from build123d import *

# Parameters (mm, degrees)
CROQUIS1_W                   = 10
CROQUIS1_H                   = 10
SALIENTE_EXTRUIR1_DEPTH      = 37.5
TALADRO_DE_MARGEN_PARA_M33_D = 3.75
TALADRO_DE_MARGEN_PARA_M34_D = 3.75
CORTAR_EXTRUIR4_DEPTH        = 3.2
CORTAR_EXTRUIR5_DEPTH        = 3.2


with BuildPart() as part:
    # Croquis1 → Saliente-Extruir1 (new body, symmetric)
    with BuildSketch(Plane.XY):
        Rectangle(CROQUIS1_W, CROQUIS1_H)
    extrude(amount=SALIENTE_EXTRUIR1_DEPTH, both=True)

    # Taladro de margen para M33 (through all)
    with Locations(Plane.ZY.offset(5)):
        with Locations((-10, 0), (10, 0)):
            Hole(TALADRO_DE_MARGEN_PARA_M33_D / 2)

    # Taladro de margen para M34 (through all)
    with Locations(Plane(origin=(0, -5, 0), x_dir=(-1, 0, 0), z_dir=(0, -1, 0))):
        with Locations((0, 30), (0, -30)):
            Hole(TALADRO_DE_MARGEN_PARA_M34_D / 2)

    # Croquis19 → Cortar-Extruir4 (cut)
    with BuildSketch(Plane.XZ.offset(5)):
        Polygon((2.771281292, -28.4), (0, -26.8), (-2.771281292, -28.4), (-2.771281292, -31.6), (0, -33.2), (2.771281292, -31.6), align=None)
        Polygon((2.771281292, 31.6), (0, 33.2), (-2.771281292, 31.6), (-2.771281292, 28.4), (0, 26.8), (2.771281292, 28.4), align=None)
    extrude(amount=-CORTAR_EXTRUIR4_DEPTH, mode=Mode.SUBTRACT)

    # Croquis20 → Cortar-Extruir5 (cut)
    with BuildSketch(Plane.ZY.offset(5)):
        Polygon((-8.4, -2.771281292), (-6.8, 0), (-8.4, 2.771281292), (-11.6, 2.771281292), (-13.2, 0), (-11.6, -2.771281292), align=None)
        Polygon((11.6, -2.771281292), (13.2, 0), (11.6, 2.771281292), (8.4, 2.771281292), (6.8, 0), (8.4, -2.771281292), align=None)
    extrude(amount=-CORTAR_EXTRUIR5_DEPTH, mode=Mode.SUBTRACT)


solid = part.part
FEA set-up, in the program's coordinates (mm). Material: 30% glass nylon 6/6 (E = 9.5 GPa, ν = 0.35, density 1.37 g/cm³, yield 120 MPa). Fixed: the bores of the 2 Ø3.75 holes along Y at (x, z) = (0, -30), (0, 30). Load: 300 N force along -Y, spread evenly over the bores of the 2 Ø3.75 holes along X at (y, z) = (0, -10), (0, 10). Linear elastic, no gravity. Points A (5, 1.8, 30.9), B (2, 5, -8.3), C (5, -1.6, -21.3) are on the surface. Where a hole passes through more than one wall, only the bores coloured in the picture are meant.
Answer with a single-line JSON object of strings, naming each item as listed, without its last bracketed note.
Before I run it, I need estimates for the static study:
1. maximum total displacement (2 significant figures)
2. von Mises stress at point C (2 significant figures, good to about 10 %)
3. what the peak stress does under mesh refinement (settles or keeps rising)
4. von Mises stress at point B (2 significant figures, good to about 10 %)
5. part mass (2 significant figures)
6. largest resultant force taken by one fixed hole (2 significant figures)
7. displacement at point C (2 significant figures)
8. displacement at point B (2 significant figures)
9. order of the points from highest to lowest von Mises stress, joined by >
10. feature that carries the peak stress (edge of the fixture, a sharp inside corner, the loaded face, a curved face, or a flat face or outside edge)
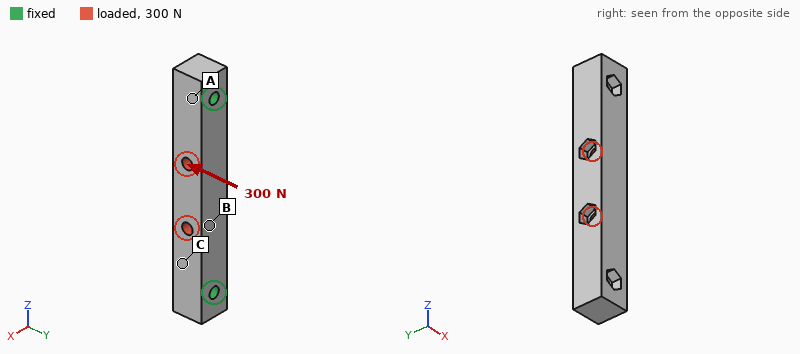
{"maximum total displacement": "60 µm", "von Mises stress at point C": "5.4 MPa", "what the peak stress does under mesh refinement": "keeps rising", "von Mises stress at point B": "8.3 MPa", "part mass": "9.4 g", "largest resultant force taken by one fixed hole": "160 N", "displacement at point C": "19 µm", "displacement at point B": "51 µm", "order of the points from highest to lowest von Mises stress, joined by >": "B > C > A", "feature that carries the peak stress": "edge of the fixture"}
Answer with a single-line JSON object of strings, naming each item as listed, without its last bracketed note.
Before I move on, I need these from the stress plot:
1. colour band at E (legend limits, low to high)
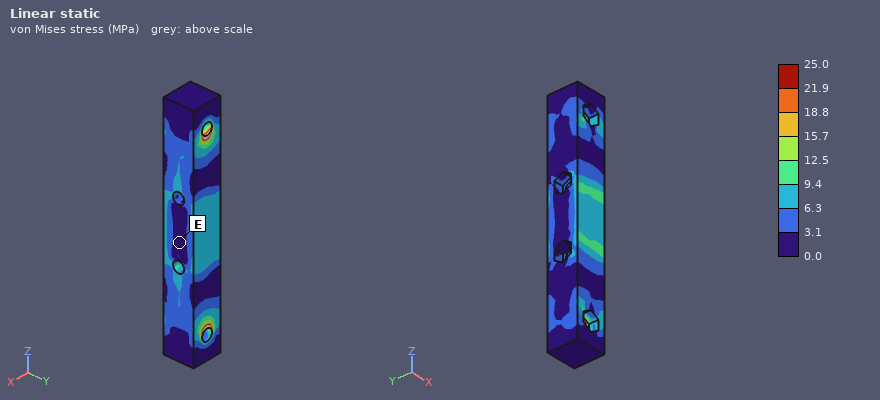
{"colour band at E": "0.0 to 3.1 MPa"}
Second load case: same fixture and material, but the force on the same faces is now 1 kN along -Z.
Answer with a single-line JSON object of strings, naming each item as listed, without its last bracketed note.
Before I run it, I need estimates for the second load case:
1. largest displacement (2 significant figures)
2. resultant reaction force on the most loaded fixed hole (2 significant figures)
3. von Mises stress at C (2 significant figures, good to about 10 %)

{"largest displacement": "16 µm", "resultant reaction force on the most loaded fixed hole": "500 N", "von Mises stress at C": "5.7 MPa"}
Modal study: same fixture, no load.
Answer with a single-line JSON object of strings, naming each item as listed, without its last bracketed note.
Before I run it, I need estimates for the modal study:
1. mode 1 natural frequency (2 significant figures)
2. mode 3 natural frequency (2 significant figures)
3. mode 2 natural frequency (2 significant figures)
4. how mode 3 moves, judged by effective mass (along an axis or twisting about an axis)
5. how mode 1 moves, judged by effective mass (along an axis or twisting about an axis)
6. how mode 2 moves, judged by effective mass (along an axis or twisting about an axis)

{"mode 1 natural frequency": "5300 Hz", "mode 3 natural frequency": "11 kHz", "mode 2 natural frequency": "5800 Hz", "how mode 3 moves, judged by effective mass": "twisting about Z", "how mode 1 moves, judged by effective mass": "along X", "how mode 2 moves, judged by effective mass": "along Y"}
